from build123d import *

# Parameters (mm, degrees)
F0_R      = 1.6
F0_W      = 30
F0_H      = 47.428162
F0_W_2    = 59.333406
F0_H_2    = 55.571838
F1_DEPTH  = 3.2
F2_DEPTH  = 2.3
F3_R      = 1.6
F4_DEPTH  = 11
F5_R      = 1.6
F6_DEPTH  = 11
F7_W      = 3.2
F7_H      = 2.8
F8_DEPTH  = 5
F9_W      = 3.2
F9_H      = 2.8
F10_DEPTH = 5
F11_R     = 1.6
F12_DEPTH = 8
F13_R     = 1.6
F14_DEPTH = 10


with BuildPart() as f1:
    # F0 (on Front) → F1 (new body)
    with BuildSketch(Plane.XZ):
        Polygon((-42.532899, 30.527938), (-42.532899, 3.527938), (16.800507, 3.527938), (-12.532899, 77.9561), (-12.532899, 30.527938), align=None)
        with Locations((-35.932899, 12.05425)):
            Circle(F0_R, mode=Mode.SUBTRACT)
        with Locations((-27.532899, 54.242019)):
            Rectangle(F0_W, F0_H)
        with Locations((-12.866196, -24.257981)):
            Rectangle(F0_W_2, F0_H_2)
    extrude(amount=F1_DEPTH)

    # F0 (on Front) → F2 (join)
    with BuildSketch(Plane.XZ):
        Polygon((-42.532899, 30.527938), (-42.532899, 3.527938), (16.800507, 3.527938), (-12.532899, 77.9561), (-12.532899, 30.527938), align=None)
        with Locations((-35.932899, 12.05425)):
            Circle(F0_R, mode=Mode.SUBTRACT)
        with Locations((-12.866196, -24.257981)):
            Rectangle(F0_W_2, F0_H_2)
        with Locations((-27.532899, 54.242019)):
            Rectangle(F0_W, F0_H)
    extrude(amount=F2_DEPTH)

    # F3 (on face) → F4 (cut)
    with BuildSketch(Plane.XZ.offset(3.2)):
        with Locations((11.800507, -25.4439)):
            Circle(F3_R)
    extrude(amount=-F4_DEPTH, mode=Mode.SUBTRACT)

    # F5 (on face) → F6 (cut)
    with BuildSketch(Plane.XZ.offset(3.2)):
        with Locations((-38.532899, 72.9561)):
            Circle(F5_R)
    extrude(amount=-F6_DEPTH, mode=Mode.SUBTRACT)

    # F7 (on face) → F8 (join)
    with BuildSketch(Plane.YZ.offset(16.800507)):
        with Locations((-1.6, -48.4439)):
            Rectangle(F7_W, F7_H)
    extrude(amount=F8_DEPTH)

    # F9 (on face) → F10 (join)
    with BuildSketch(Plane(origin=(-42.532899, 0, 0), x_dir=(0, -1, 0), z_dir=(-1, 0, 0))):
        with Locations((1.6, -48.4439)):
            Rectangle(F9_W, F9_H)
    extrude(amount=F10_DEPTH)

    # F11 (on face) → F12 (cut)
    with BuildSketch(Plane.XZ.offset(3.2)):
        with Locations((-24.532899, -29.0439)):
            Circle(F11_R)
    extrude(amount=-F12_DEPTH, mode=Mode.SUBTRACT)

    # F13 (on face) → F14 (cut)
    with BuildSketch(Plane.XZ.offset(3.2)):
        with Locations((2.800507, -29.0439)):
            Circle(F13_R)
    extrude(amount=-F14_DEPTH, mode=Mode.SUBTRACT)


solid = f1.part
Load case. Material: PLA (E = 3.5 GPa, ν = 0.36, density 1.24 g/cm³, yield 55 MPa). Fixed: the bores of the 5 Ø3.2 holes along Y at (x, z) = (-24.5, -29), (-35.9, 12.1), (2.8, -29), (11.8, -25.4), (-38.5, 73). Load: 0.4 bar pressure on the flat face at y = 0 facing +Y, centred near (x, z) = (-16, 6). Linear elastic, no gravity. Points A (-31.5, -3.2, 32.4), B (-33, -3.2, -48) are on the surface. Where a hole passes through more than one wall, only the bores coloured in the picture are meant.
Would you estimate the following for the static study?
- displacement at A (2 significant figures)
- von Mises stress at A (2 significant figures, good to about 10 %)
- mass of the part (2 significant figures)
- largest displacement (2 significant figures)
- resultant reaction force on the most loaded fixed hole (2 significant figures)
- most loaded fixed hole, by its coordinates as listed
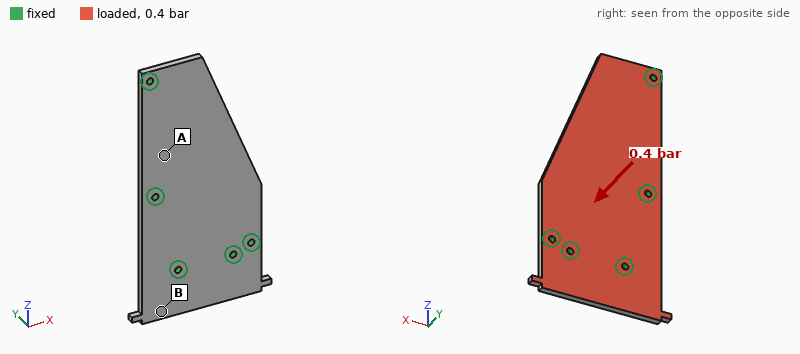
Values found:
0.31 mm
5.0 MPa
26 g
1.6 mm
86 N
(-35.9, 12.1)
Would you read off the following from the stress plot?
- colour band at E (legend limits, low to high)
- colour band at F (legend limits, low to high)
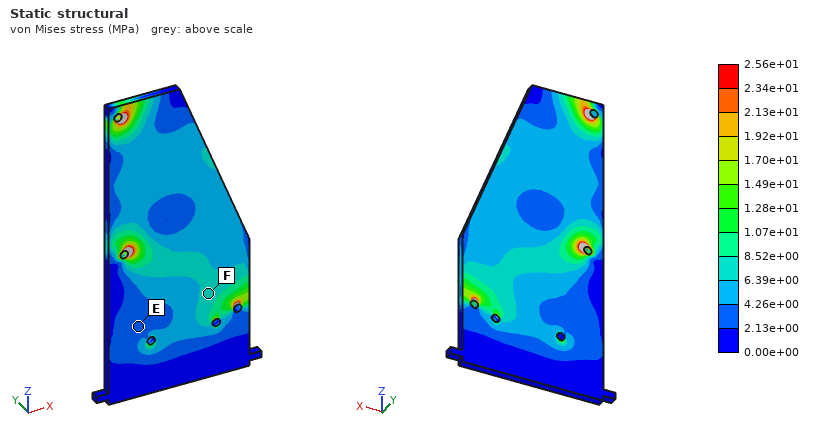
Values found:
2.13e+00 to 4.26e+00 MPa
6.39e+00 to 8.52e+00 MPa
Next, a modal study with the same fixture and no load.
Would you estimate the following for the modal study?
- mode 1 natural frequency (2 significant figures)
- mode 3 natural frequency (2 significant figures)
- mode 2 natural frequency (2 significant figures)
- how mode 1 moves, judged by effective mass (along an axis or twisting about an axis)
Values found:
540 Hz
1400 Hz
1100 Hz
along Y
